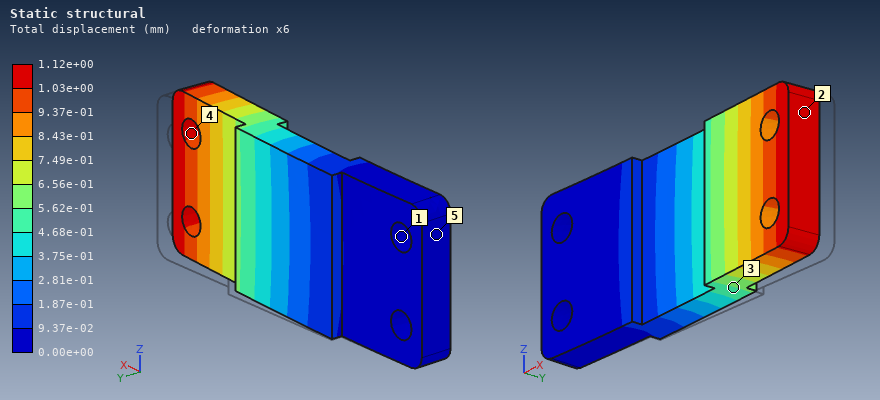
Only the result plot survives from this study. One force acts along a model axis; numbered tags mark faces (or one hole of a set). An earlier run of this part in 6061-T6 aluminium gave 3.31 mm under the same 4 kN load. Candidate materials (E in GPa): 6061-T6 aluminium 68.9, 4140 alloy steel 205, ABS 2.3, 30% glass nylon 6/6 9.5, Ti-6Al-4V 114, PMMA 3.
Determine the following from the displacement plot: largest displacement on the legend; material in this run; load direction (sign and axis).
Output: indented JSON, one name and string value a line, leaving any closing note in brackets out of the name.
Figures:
{
  "largest displacement on the legend": "1.12e+00 mm",
  "material in this run": "4140 alloy steel",
  "load direction": "-Y"
}
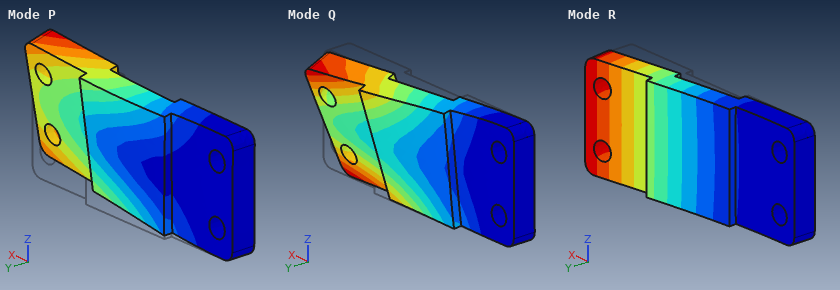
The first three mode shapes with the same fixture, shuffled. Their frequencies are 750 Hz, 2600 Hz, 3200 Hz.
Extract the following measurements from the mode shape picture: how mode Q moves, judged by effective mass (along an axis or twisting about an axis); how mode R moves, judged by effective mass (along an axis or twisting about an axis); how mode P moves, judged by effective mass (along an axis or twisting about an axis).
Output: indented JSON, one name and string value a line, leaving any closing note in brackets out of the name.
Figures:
{
  "how mode Q moves, judged by effective mass": "along Z",
  "how mode R moves, judged by effective mass": "along Y",
  "how mode P moves, judged by effective mass": "along Z"
}
